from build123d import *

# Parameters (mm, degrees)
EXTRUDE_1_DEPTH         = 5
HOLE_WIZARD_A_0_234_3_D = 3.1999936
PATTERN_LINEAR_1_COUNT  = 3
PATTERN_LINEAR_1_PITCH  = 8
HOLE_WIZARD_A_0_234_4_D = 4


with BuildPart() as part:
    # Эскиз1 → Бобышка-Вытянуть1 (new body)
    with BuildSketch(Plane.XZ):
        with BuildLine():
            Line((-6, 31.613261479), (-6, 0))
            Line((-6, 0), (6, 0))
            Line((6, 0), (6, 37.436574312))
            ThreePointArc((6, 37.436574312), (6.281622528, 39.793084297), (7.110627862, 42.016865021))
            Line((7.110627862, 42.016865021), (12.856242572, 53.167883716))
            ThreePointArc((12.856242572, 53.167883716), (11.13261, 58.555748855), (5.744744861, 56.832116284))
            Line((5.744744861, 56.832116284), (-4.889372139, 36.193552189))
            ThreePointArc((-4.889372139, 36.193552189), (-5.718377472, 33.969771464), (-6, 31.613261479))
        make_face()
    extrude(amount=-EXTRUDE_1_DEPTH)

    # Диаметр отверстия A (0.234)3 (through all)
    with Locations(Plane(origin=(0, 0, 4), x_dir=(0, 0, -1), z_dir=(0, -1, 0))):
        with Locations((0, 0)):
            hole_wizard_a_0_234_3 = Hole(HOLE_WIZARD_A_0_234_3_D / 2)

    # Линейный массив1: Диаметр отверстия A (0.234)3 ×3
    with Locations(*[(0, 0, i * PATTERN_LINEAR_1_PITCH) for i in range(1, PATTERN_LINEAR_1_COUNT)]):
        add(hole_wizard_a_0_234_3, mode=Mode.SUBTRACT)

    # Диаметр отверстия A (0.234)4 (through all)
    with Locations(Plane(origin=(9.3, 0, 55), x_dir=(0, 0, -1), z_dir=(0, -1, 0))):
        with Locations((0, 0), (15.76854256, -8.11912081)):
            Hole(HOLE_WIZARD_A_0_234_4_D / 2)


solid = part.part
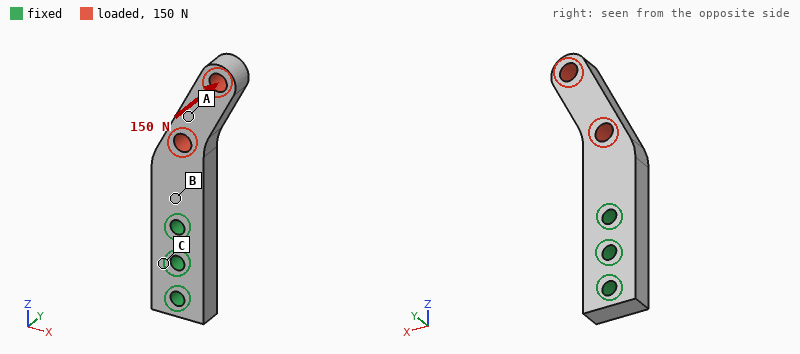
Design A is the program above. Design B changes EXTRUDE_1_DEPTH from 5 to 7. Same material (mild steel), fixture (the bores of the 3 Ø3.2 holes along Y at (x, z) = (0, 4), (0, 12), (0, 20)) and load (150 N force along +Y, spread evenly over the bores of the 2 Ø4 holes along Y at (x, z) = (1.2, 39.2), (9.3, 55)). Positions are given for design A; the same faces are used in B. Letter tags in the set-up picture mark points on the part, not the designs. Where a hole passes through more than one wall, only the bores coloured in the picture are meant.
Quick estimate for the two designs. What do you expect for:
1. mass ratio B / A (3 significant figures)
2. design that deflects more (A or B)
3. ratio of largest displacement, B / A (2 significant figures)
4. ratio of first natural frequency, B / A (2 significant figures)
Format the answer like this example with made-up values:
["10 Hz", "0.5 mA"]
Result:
["1.40", "A", "0.38", "1.4"]
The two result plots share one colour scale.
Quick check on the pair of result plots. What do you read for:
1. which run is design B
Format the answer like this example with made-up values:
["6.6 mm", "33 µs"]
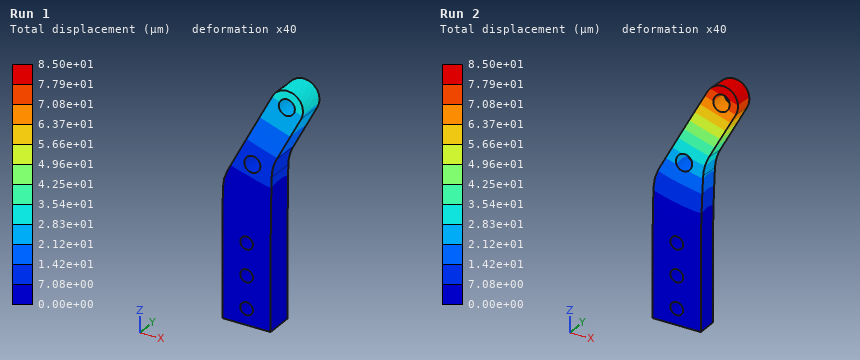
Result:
["Run 1"]
